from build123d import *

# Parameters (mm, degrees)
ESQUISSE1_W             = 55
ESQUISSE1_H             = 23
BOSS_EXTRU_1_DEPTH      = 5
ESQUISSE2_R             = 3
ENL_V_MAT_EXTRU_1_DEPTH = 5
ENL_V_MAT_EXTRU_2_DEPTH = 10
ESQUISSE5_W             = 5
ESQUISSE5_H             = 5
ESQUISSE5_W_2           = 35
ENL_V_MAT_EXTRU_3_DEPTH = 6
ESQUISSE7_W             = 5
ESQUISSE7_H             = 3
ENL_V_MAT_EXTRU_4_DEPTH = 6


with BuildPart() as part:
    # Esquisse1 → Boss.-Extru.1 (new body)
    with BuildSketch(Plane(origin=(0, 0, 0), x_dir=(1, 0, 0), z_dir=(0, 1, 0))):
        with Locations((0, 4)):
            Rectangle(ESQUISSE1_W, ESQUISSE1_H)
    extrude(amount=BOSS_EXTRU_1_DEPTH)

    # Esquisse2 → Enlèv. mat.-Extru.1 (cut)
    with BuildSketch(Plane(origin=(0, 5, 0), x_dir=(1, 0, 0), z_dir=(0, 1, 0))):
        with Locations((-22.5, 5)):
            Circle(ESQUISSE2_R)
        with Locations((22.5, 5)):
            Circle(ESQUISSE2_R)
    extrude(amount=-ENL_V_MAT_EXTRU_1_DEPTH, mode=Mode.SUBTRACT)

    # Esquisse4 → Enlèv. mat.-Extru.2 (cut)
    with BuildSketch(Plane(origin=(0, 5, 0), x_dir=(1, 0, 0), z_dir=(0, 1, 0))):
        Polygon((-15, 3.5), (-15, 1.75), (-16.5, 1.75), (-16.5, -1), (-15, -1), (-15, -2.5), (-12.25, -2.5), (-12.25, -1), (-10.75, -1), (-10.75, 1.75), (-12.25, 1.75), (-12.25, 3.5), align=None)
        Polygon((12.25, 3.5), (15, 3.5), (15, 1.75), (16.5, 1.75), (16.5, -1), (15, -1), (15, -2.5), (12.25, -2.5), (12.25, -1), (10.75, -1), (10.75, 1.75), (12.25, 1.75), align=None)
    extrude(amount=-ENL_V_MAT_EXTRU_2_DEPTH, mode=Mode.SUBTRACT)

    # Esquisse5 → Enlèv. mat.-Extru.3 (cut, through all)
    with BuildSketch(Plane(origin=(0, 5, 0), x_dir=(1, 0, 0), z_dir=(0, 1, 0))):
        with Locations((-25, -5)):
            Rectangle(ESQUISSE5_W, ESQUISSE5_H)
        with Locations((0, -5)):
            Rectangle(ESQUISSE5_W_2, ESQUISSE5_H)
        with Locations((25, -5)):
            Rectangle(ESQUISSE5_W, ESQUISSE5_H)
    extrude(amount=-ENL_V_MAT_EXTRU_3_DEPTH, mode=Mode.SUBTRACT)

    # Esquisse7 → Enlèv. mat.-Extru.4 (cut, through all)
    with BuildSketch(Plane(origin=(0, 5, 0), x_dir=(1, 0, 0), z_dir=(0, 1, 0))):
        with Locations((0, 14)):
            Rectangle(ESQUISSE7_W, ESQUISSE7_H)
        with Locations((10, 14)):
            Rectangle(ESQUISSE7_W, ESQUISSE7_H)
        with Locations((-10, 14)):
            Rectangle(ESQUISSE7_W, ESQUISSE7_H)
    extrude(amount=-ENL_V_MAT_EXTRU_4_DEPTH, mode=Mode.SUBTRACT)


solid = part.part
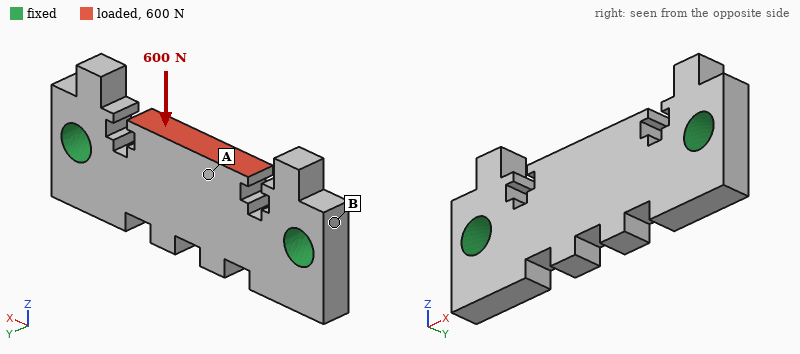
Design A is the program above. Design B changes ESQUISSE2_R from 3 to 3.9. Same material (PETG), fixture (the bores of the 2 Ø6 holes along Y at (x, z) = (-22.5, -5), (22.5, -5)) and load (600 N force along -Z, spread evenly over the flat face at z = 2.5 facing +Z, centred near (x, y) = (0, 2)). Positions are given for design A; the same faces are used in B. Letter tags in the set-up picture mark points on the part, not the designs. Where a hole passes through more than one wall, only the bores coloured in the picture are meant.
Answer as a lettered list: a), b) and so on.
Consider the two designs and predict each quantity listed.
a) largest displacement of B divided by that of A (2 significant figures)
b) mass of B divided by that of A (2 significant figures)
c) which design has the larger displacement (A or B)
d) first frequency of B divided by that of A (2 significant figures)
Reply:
a) 0.87
b) 0.96
c) A
d) 1.1
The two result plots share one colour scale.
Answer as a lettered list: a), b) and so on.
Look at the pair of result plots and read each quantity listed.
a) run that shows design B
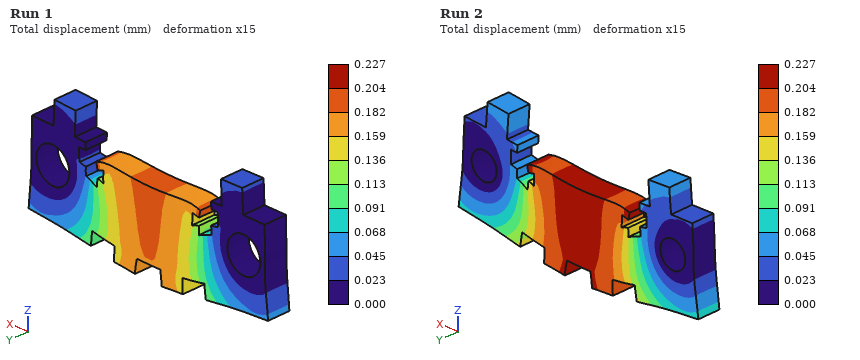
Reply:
a) Run 1
